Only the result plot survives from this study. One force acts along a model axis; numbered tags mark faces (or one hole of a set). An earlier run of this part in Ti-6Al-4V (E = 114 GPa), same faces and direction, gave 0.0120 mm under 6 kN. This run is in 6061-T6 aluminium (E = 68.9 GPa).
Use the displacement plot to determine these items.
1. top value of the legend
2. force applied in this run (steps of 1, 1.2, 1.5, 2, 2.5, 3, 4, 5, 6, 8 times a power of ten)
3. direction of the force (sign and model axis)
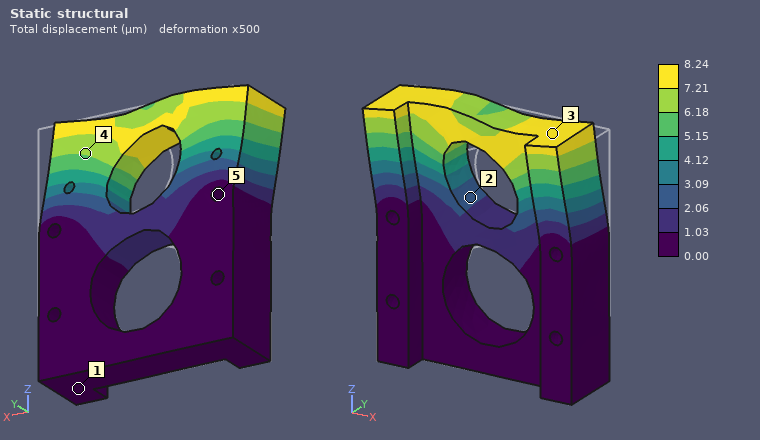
8.24 µm
2.5 kN
-X
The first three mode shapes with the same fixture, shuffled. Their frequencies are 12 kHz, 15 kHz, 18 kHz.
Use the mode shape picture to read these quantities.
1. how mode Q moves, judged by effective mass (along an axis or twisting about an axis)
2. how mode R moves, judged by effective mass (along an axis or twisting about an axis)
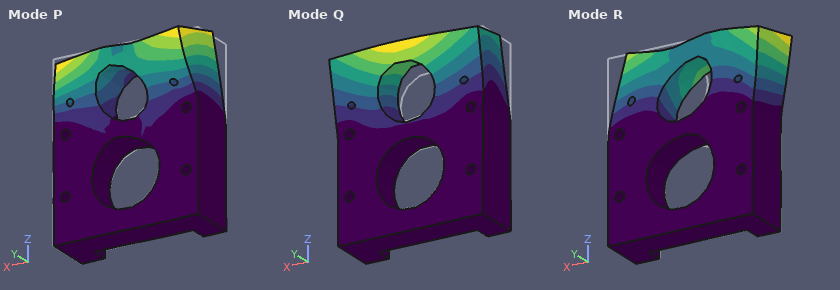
along Y
along X
